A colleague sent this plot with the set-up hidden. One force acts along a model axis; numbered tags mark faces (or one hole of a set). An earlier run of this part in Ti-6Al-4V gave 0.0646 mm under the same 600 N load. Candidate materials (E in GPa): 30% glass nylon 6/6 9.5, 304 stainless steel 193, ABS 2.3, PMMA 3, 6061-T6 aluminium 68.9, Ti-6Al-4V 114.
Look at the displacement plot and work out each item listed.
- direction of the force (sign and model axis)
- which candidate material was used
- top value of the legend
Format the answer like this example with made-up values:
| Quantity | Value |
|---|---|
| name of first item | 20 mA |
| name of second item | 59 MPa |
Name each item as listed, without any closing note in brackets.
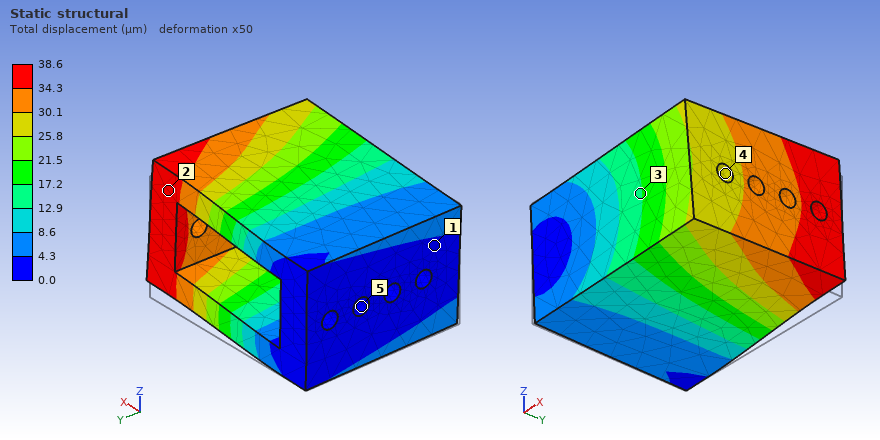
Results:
| Quantity | Value |
|---|---|
| direction of the force | +Z |
| which candidate material was used | 304 stainless steel |
| top value of the legend | 38.6 µm |
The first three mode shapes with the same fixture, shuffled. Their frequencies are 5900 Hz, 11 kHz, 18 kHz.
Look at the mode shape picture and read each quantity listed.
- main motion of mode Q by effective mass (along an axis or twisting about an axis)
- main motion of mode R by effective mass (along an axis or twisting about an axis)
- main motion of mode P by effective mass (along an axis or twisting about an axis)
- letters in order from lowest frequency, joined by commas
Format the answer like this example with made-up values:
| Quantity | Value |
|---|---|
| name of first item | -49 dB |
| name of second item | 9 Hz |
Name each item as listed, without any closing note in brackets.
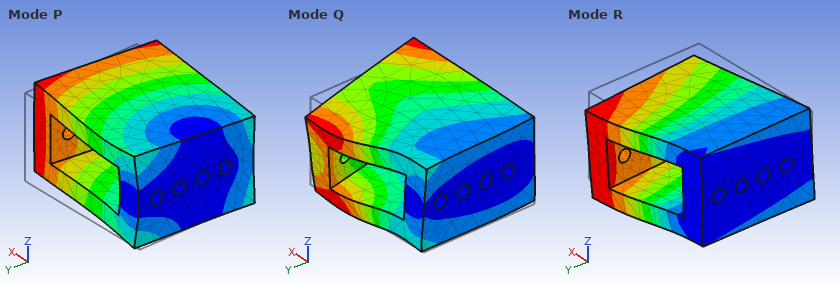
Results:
| Quantity | Value |
|---|---|
| main motion of mode Q by effective mass | twisting about X |
| main motion of mode R by effective mass | along Z |
| main motion of mode P by effective mass | along Y |
| letters in order from lowest frequency, joined by commas | R, P, Q |
